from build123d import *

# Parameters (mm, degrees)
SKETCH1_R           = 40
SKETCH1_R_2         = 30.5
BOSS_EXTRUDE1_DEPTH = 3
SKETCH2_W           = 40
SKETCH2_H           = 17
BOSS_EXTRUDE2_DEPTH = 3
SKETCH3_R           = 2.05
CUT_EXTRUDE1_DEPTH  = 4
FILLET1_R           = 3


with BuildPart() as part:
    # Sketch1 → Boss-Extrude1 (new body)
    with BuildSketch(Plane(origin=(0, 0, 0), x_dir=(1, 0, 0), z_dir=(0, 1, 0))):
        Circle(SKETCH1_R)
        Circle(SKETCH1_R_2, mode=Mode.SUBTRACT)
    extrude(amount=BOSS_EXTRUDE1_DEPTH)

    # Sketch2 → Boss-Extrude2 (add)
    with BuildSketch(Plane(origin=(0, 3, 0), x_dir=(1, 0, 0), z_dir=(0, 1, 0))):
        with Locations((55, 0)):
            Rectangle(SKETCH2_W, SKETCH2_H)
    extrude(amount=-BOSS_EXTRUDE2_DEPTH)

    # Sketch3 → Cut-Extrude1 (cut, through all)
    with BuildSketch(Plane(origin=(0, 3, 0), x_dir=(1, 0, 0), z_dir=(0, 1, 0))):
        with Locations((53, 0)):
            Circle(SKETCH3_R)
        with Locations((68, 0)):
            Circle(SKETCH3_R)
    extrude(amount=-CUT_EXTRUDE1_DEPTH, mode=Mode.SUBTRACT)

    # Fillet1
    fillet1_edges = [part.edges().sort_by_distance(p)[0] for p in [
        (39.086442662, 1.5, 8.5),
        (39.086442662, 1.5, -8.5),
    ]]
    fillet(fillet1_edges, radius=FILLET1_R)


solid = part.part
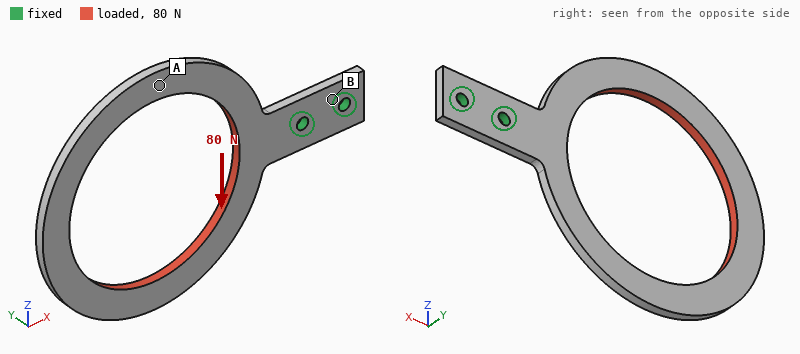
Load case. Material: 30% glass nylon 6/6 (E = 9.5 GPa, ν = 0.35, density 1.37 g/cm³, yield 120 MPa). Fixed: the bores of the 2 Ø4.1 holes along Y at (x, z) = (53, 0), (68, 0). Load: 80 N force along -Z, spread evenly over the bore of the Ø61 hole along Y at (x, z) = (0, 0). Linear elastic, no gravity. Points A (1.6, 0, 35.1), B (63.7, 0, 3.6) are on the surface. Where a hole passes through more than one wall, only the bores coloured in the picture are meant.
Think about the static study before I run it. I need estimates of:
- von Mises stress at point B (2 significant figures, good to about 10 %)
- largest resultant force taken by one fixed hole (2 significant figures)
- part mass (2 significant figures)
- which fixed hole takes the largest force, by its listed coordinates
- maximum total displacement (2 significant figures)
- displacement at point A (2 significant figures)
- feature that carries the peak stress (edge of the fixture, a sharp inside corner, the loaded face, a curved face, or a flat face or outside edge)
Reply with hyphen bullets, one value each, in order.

- 8.8 MPa
- 250 N
- 11 g
- (53, 0)
- 1.5 mm
- 0.92 mm
- edge of the fixture
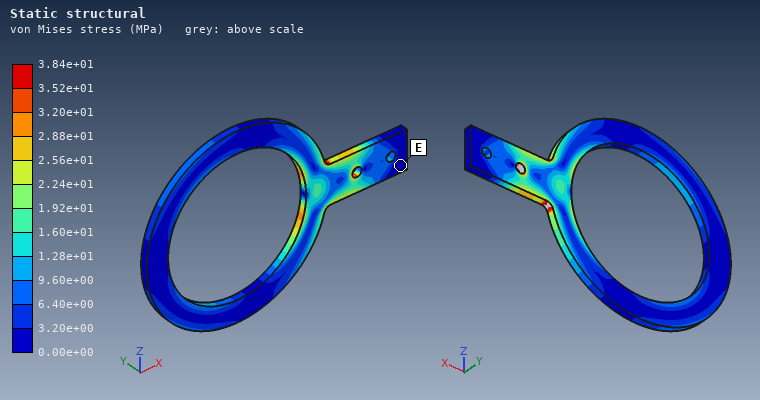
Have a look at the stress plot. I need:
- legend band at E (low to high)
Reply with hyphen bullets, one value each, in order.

- 0.00e+00 to 3.20e+00 MPa
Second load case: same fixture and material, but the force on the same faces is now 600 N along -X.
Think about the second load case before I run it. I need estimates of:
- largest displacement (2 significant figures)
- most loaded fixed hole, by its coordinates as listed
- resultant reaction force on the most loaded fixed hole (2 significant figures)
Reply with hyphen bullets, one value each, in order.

- 0.85 mm
- (53, 0)
- 510 N
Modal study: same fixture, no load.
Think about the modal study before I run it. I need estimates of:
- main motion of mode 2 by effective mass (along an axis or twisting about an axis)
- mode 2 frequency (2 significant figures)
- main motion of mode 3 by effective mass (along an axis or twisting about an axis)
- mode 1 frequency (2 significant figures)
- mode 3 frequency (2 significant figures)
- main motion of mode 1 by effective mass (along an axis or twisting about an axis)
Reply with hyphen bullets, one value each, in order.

- twisting about X
- 240 Hz
- along Z
- 110 Hz
- 430 Hz
- along Y
